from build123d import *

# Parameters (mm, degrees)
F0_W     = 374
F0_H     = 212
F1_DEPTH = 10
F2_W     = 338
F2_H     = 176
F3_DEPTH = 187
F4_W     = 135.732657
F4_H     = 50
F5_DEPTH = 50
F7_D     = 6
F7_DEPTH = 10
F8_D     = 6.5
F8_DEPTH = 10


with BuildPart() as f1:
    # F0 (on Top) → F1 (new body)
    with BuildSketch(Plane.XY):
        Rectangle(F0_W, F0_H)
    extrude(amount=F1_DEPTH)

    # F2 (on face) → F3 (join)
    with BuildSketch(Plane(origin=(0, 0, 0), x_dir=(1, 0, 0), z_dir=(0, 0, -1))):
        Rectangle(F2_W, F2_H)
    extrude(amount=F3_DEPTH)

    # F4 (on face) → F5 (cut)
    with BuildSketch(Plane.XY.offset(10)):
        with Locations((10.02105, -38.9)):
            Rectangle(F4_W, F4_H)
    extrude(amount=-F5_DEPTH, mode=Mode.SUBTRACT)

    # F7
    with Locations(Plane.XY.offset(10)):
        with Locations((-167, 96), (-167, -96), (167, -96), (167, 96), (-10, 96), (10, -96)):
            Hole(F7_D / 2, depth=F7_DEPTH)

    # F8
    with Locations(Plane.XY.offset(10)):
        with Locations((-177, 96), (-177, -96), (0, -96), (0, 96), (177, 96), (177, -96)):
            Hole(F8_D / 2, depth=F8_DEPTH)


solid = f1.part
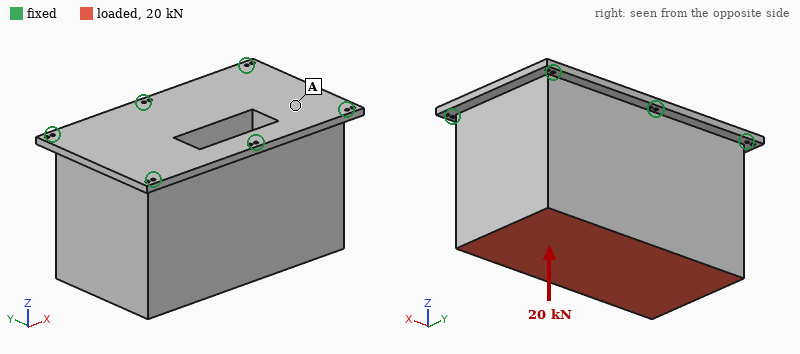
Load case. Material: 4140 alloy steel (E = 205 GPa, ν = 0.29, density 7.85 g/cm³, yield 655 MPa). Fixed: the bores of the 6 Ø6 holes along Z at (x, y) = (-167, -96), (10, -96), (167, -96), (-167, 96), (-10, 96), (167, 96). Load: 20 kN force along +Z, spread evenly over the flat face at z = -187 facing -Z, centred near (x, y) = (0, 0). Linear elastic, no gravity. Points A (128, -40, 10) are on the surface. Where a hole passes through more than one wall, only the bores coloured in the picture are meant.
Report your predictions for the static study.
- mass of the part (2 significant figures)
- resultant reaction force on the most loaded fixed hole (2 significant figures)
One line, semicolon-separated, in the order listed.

91 kg; 4.6 kN
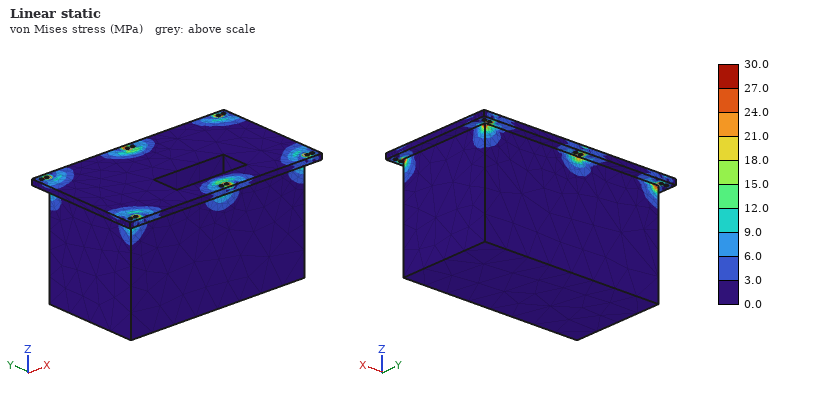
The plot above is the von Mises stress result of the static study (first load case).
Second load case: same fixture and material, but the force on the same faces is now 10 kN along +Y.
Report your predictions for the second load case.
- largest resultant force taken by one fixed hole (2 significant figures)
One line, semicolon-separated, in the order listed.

5.0 kN
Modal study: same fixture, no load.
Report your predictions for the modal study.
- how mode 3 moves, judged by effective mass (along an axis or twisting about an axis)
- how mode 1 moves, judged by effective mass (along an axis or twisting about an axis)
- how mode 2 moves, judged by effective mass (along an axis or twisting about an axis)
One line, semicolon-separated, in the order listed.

along Z; along Y; along X
